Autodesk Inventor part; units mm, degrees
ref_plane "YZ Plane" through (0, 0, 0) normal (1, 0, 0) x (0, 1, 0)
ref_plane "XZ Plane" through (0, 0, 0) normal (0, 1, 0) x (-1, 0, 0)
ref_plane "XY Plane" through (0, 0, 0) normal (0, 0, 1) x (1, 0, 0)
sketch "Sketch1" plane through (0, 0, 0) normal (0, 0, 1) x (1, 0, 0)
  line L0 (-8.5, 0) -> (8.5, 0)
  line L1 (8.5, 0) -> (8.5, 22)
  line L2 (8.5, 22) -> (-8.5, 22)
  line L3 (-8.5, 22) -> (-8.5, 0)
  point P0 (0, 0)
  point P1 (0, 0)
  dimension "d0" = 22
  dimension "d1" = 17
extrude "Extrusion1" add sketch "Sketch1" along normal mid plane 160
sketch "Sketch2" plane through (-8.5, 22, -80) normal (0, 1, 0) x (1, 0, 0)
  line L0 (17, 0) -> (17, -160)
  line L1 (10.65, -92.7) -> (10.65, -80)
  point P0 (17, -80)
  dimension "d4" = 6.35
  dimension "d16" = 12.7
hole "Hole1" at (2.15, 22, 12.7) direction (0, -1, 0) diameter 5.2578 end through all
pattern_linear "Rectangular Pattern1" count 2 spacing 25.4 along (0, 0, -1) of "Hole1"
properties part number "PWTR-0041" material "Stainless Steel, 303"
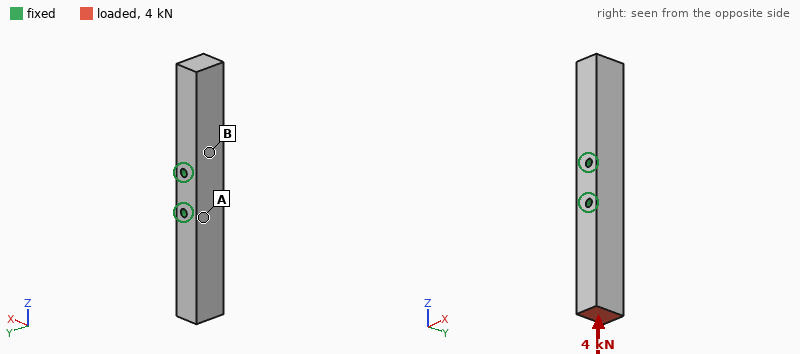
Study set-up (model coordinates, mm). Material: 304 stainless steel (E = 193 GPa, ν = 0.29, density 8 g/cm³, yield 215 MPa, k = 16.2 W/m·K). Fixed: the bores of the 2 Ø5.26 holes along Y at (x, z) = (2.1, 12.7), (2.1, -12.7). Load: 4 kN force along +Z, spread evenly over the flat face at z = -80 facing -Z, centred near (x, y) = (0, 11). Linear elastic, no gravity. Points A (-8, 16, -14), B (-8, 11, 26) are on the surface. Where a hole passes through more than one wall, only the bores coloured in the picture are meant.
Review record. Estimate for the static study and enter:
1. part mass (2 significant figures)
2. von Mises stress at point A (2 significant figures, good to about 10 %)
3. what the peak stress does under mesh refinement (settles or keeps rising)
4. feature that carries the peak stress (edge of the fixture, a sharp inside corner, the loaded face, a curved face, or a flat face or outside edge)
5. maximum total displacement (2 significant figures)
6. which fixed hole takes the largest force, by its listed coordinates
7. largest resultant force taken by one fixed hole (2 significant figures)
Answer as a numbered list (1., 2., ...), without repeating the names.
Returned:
1. 470 g
2. 8.2 MPa
3. keeps rising
4. edge of the fixture
5. 4.9 µm
6. (2.1, -12.7)
7. 3.6 kN
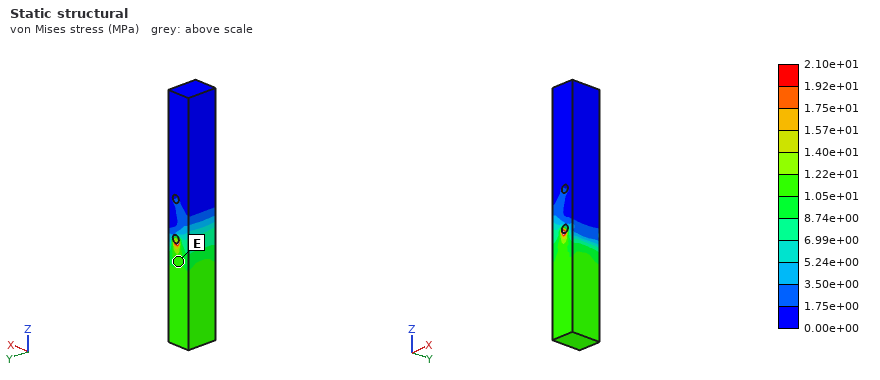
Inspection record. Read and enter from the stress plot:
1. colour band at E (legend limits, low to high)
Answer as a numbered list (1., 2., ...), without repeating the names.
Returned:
1. 1.05e+01 to 1.22e+01 MPa
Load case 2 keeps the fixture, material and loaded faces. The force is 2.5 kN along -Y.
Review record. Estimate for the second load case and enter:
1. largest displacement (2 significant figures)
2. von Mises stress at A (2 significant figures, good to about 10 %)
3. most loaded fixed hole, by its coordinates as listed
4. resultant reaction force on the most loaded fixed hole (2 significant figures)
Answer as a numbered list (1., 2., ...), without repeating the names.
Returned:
1. 99 µm
2. 34 MPa
3. (2.1, -12.7)
4. 3.3 kN
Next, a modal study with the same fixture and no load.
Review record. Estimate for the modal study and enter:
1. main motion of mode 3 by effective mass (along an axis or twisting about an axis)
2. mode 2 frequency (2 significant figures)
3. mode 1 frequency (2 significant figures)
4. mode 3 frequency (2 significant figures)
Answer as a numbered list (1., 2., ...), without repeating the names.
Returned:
1. twisting about X
2. 2600 Hz
3. 2500 Hz
4. 3500 Hz
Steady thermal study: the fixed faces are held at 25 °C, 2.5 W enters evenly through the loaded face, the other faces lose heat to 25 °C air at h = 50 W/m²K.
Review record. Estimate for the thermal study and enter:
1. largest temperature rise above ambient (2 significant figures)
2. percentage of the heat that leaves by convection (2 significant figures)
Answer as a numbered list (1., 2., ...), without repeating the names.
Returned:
1. 15 K
2. 65 %
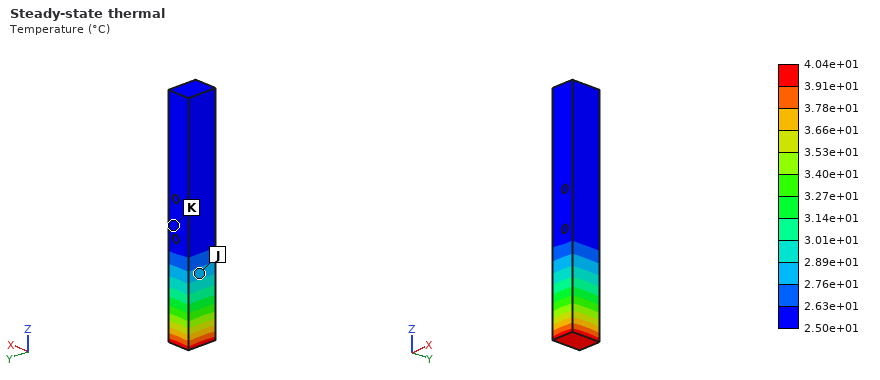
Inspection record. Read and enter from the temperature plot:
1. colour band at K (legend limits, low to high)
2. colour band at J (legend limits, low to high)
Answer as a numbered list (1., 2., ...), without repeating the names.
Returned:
1. 2.50e+01 to 2.63e+01 °C
2. 2.76e+01 to 2.89e+01 °C
